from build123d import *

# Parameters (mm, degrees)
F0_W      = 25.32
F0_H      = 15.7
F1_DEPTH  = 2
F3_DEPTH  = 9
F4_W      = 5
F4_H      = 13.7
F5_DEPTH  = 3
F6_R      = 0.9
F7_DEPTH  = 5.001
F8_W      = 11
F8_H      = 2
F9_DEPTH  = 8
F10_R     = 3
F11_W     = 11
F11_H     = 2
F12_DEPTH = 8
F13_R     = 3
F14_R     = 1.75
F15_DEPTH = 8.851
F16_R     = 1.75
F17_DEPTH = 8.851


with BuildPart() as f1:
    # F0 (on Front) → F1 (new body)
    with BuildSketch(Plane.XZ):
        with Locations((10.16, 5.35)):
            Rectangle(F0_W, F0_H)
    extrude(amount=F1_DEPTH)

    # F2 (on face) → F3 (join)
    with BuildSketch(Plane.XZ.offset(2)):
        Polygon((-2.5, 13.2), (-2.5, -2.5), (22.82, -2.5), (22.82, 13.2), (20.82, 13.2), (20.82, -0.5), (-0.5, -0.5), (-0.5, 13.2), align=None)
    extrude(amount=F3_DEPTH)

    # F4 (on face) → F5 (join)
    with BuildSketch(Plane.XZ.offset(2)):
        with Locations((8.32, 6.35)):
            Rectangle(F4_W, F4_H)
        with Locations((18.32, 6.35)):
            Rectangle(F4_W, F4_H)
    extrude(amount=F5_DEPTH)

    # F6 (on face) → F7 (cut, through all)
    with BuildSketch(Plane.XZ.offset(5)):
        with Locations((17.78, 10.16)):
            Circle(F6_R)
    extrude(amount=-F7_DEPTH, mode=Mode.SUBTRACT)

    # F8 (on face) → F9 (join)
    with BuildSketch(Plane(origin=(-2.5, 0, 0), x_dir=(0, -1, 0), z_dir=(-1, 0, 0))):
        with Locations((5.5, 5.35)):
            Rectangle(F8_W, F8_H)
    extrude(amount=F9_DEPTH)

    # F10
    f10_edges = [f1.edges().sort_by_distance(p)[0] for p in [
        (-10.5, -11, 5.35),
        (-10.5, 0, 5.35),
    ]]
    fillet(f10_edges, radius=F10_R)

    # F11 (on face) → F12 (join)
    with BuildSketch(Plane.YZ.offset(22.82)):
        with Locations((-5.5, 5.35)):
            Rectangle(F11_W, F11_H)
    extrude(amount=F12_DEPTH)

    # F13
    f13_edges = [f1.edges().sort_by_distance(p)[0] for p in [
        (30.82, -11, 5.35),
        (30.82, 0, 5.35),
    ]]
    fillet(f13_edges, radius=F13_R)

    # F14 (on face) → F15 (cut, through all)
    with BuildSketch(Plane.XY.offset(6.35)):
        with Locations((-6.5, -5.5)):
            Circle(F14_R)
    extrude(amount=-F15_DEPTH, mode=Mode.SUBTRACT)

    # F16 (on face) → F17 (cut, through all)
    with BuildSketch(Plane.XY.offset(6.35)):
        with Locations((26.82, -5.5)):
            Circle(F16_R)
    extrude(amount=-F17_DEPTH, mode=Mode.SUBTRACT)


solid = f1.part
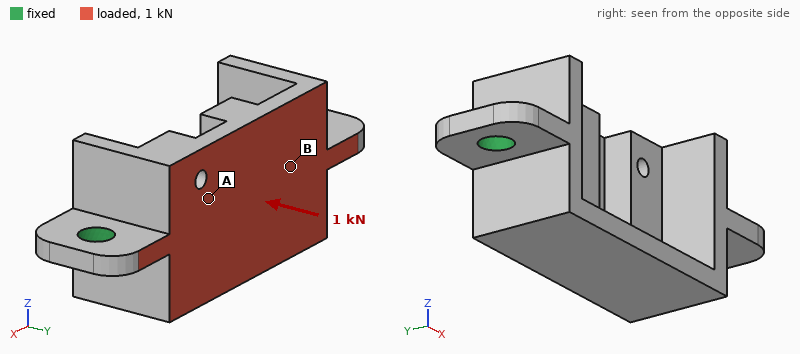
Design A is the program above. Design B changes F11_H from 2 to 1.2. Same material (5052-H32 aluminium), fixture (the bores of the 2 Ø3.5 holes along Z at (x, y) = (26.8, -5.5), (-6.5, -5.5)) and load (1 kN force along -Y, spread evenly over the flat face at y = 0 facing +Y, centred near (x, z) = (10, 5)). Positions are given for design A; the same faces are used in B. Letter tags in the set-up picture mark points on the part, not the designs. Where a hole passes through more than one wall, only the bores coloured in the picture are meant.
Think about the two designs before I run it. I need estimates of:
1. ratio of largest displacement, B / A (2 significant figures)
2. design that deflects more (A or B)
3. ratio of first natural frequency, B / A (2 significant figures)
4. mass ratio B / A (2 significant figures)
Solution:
1.2
B
0.77
0.98
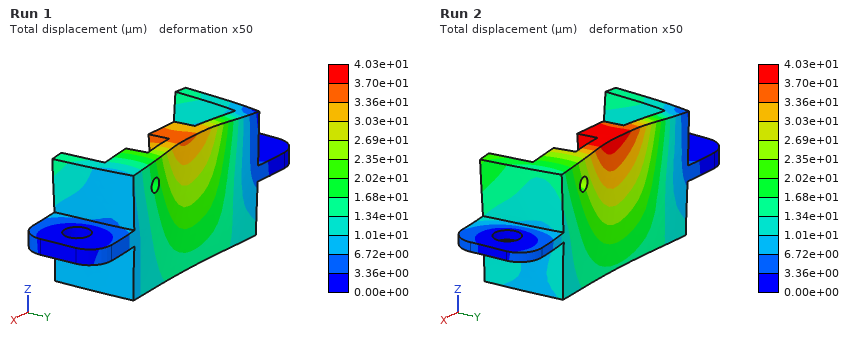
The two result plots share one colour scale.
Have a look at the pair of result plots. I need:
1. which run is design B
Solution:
Run 2
